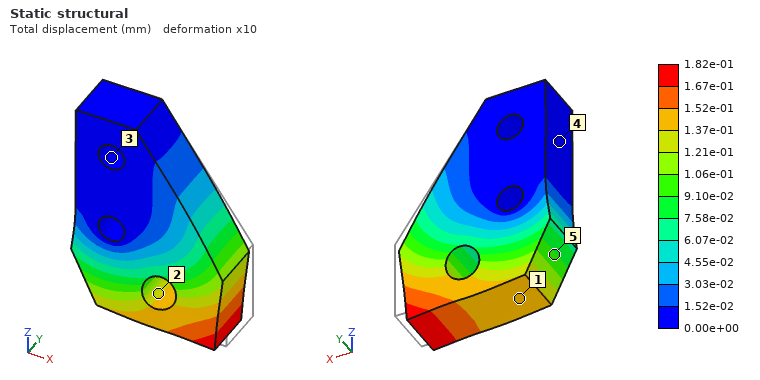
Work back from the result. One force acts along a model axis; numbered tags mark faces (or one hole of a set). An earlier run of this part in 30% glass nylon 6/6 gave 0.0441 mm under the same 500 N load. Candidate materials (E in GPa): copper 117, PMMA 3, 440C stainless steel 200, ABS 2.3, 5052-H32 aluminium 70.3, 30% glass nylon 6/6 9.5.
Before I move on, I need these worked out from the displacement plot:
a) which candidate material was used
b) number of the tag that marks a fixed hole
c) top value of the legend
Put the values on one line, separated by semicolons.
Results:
ABS; 3; 1.82e-01 mm
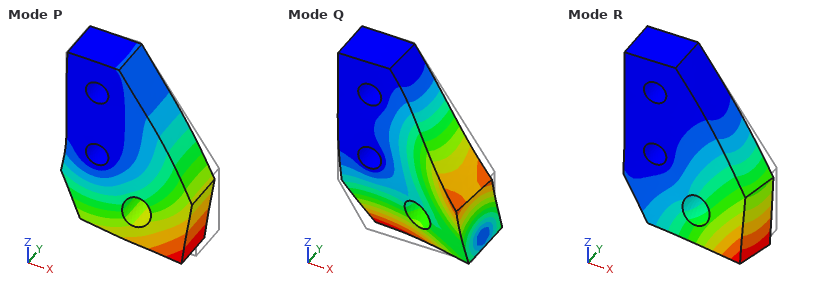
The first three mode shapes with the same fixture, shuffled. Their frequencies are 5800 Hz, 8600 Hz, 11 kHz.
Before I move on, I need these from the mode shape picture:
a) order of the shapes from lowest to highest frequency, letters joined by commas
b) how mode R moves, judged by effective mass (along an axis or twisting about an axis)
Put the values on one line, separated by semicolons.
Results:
R, P, Q; along Y
